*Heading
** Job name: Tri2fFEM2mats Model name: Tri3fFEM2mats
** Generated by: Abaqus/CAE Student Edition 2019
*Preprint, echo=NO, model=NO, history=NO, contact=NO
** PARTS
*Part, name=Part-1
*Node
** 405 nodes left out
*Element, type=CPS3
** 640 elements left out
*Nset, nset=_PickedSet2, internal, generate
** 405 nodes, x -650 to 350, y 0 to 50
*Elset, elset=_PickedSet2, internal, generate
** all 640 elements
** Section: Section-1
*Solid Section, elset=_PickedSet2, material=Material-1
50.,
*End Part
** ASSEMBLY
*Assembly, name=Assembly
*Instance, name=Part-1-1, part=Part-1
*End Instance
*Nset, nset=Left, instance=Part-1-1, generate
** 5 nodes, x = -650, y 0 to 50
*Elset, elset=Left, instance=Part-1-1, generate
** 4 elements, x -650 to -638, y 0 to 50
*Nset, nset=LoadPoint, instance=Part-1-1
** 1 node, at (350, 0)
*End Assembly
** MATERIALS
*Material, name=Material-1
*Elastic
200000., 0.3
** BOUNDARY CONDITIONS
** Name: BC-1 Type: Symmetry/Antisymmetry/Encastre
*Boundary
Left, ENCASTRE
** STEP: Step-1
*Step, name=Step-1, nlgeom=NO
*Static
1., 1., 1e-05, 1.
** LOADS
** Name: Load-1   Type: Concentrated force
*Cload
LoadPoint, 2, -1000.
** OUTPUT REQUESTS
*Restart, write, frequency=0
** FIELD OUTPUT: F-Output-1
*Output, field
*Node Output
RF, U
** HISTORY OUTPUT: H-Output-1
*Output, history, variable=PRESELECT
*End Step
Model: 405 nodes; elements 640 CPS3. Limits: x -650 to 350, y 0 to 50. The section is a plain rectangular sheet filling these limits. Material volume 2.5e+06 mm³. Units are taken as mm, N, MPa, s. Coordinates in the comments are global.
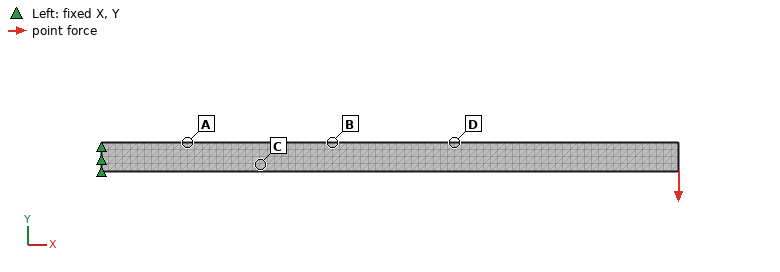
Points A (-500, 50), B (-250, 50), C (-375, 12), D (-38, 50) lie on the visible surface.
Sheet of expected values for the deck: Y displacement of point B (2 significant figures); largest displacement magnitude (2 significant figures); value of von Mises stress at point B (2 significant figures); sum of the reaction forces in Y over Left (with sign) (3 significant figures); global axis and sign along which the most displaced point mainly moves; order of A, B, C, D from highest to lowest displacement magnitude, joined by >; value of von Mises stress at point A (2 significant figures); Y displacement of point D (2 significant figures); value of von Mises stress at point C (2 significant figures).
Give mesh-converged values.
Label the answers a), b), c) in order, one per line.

a) -0.65 mm
b) 3.1 mm
c) 28 MPa
d) 1000 N
e) -Y
f) D > B > C > A
g) 39 MPa
h) -1.4 mm
i) 17 MPa
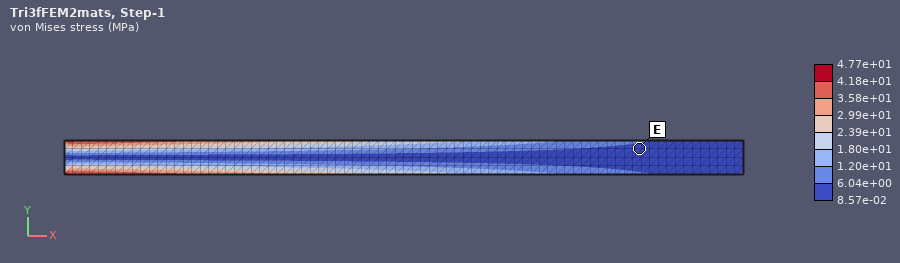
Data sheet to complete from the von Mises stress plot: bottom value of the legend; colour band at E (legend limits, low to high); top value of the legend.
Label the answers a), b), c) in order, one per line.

a) 8.57e-02 MPa
b) 8.57e-02 to 6.04e+00 MPa
c) 4.77e+01 MPa
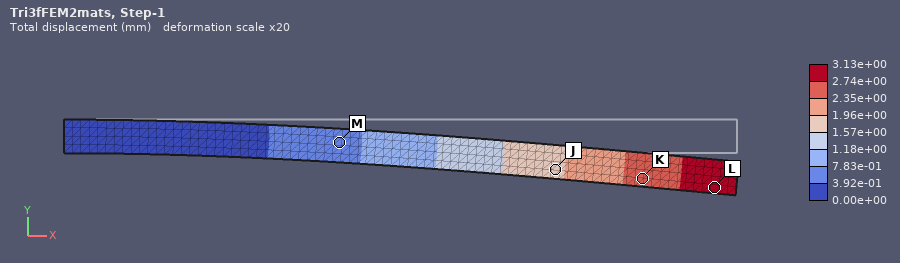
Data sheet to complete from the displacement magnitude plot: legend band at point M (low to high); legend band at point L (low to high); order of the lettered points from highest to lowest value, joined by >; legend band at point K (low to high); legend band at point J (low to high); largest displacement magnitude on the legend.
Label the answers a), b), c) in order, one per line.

a) 3.92e-01 to 7.83e-01 mm
b) 2.74e+00 to 3.13e+00 mm
c) L > K > J > M
d) 2.35e+00 to 2.74e+00 mm
e) 1.57e+00 to 1.96e+00 mm
f) 3.13e+00 mm
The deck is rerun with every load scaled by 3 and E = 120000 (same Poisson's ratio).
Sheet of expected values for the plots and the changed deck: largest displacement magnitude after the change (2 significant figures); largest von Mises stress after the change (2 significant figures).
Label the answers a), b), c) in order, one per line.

a) 16 mm
b) 140 MPa
